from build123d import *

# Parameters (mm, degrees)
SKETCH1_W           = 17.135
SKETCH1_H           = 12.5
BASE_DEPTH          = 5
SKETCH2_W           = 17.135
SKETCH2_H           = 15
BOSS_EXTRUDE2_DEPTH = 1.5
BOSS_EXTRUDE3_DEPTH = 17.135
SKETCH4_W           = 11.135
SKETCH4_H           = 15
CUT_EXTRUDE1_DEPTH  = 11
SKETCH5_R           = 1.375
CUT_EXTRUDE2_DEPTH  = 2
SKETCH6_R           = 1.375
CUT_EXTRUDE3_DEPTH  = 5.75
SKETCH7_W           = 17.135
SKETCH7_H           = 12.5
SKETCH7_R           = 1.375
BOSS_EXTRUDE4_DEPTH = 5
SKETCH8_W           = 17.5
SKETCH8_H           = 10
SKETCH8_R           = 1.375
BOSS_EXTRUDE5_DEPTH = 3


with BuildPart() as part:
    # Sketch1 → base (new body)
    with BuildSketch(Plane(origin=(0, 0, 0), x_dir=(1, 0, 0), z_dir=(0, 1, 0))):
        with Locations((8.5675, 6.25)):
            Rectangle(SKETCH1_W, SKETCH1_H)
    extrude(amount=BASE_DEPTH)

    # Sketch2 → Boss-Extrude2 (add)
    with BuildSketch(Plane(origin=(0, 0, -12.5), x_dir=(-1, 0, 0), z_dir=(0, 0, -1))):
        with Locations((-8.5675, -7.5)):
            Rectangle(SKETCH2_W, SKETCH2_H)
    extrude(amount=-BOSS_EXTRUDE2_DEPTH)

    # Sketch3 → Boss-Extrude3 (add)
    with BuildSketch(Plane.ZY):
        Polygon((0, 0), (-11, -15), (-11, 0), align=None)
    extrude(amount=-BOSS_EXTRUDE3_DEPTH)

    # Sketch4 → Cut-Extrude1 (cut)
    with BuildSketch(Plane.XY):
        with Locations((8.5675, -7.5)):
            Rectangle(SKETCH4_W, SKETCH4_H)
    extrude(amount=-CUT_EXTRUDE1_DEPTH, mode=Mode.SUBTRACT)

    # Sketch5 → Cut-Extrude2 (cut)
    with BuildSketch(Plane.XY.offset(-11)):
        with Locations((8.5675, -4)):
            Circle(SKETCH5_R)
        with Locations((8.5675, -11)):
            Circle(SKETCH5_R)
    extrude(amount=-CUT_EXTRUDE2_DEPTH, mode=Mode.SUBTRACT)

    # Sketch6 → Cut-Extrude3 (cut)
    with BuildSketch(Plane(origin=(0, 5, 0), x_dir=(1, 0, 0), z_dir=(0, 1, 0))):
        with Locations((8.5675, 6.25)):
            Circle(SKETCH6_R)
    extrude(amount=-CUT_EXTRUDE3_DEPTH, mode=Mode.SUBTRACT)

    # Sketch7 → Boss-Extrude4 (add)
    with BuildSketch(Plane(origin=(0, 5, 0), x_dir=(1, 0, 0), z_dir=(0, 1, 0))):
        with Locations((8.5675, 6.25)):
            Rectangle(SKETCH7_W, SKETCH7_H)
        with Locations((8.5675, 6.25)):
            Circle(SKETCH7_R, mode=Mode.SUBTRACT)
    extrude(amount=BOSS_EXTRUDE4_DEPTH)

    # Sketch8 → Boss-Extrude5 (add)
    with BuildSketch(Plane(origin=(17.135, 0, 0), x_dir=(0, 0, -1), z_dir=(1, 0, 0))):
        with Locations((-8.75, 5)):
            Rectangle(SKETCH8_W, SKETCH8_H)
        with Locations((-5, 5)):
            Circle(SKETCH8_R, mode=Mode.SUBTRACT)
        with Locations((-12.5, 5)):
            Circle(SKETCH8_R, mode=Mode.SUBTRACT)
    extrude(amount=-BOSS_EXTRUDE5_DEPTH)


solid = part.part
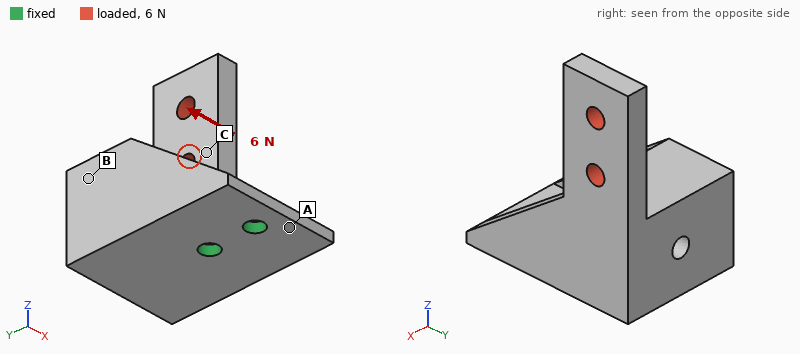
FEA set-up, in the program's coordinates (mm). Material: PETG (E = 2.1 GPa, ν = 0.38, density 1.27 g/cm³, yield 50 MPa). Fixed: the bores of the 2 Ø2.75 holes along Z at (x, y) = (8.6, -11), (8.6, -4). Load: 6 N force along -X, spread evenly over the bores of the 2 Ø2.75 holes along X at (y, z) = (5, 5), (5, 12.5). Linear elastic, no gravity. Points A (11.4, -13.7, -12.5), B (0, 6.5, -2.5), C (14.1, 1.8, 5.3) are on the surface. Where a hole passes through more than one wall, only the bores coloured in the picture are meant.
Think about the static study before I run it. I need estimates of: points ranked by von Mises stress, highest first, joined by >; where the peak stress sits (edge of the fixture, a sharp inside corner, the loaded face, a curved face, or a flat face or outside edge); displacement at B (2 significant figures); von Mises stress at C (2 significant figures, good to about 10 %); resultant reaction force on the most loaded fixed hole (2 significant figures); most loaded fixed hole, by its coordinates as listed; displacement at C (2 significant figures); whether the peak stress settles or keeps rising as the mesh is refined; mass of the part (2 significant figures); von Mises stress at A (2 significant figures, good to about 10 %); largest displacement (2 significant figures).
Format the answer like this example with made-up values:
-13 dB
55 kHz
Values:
A > C > B
edge of the fixture
0.14 mm
1.9 MPa
11 N
(8.6, -4)
0.22 mm
keeps rising
4.4 g
3.9 MPa
0.45 mm
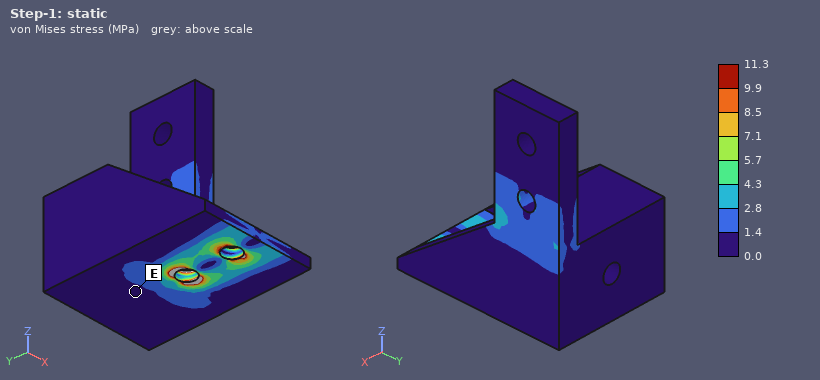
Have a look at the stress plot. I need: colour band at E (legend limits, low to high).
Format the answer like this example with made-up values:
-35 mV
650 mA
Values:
0.0 to 1.4 MPa
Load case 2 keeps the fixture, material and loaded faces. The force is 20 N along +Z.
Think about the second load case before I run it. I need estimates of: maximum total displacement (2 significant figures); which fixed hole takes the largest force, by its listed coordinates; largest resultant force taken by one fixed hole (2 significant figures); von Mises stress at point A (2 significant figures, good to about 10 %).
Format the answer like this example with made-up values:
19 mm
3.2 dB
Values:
0.51 mm
(8.6, -4)
34 N
2.6 MPa
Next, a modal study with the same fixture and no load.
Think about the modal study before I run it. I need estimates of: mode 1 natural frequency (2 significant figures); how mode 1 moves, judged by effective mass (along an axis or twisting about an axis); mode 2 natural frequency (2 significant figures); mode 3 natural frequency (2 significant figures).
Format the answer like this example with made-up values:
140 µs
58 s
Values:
690 Hz
along X
870 Hz
2300 Hz
